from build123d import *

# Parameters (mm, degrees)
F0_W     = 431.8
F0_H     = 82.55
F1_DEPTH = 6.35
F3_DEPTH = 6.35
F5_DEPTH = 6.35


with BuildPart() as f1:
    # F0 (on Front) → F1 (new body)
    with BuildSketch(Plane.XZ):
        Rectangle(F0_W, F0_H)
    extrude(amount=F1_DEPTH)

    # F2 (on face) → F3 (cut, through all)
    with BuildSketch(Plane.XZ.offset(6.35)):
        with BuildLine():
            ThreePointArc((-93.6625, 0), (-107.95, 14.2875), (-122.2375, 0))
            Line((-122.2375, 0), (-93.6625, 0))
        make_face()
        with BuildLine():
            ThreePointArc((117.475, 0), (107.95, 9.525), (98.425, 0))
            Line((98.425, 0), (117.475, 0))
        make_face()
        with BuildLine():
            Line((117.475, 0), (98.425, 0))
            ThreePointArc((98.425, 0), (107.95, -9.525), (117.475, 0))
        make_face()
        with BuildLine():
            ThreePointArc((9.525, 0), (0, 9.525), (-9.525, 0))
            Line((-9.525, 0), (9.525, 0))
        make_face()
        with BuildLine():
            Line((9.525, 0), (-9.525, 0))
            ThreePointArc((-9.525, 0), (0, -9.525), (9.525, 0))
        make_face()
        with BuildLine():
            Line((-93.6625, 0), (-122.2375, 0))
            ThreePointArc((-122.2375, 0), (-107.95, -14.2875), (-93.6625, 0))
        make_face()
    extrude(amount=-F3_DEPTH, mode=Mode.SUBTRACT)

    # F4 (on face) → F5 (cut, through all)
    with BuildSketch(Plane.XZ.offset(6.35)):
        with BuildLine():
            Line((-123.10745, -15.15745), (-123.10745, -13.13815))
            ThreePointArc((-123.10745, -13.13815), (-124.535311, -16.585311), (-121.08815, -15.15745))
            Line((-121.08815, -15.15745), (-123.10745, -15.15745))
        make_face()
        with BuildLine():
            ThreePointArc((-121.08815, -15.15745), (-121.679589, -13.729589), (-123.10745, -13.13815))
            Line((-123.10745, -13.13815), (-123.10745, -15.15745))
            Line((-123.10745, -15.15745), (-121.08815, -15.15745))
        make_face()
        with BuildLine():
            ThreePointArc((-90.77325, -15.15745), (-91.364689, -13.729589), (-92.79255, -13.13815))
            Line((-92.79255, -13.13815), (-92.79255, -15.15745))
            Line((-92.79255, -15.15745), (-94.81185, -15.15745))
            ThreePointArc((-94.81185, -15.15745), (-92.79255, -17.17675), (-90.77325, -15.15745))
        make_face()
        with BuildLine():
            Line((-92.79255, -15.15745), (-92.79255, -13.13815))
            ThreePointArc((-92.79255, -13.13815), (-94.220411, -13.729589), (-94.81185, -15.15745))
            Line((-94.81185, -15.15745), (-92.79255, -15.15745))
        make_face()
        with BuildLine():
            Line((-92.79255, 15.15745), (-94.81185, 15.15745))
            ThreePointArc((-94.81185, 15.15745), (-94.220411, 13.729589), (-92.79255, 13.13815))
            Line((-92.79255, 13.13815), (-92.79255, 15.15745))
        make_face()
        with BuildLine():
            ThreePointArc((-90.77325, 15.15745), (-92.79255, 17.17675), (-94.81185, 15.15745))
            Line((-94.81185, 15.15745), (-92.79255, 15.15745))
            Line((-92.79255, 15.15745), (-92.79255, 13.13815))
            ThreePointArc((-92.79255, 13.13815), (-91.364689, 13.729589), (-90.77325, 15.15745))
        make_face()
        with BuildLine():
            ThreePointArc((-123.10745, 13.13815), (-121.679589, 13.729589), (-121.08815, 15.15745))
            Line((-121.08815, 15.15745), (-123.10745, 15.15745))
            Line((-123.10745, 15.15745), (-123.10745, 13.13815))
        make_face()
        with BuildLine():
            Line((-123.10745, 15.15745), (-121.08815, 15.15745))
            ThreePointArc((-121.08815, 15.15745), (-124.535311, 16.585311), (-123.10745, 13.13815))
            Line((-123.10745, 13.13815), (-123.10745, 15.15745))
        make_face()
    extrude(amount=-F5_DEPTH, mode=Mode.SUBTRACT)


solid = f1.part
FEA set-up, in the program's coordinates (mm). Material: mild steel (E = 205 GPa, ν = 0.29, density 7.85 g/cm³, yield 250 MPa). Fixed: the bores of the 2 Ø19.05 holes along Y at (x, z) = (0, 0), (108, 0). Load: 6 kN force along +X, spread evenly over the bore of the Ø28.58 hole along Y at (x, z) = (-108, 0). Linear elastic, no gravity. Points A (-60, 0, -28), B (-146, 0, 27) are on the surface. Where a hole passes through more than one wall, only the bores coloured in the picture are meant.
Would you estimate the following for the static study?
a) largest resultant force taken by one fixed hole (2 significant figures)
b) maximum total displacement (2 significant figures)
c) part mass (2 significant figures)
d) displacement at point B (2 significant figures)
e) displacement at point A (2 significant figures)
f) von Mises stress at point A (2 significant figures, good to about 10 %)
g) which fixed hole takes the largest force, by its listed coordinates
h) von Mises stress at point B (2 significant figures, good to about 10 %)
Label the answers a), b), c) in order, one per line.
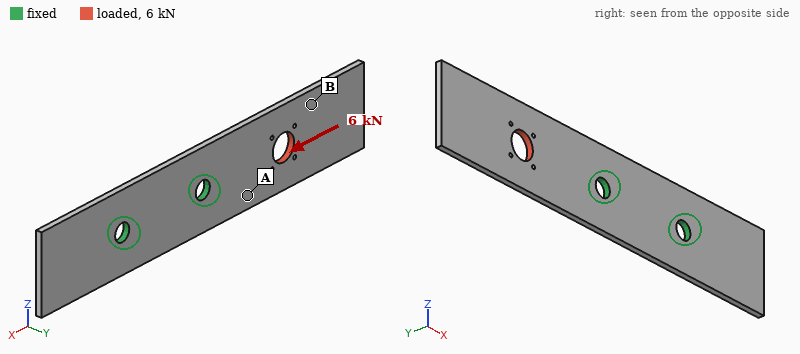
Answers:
a) 5.3 kN
b) 8.8 µm
c) 1.7 kg
d) 7.4 µm
e) 4.1 µm
f) 11 MPa
g) (0, 0)
h) 3.5 MPa
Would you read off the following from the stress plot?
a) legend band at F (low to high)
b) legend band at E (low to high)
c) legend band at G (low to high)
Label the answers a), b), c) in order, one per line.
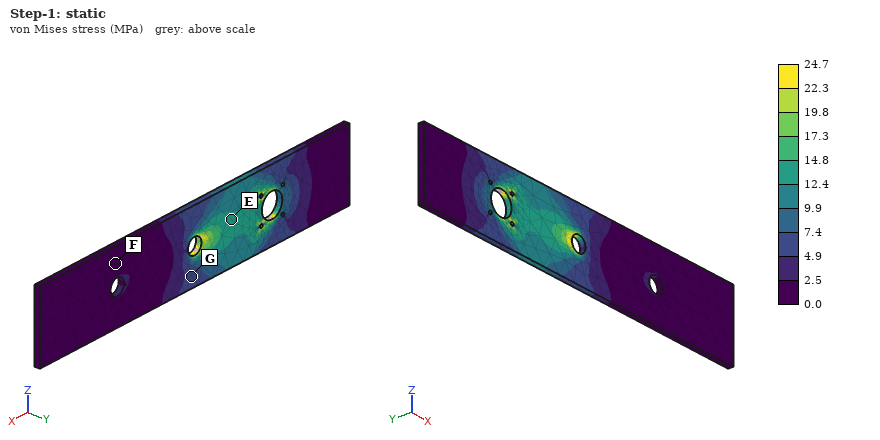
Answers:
a) 0.0 to 2.5 MPa
b) 12.4 to 14.8 MPa
c) 4.9 to 7.4 MPa
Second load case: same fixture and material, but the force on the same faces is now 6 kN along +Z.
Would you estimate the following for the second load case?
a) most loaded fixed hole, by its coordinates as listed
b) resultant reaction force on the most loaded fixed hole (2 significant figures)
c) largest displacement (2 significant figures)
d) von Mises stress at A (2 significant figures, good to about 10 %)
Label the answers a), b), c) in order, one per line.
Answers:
a) (0, 0)
b) 9.9 kN
c) 0.21 mm
d) 30 MPa
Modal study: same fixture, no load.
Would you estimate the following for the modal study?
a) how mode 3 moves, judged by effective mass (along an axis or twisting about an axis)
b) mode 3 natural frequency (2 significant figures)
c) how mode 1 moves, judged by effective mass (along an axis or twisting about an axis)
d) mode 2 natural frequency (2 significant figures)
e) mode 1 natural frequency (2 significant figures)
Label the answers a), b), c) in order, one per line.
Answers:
a) twisting about X
b) 560 Hz
c) along Y
d) 490 Hz
e) 120 Hz
